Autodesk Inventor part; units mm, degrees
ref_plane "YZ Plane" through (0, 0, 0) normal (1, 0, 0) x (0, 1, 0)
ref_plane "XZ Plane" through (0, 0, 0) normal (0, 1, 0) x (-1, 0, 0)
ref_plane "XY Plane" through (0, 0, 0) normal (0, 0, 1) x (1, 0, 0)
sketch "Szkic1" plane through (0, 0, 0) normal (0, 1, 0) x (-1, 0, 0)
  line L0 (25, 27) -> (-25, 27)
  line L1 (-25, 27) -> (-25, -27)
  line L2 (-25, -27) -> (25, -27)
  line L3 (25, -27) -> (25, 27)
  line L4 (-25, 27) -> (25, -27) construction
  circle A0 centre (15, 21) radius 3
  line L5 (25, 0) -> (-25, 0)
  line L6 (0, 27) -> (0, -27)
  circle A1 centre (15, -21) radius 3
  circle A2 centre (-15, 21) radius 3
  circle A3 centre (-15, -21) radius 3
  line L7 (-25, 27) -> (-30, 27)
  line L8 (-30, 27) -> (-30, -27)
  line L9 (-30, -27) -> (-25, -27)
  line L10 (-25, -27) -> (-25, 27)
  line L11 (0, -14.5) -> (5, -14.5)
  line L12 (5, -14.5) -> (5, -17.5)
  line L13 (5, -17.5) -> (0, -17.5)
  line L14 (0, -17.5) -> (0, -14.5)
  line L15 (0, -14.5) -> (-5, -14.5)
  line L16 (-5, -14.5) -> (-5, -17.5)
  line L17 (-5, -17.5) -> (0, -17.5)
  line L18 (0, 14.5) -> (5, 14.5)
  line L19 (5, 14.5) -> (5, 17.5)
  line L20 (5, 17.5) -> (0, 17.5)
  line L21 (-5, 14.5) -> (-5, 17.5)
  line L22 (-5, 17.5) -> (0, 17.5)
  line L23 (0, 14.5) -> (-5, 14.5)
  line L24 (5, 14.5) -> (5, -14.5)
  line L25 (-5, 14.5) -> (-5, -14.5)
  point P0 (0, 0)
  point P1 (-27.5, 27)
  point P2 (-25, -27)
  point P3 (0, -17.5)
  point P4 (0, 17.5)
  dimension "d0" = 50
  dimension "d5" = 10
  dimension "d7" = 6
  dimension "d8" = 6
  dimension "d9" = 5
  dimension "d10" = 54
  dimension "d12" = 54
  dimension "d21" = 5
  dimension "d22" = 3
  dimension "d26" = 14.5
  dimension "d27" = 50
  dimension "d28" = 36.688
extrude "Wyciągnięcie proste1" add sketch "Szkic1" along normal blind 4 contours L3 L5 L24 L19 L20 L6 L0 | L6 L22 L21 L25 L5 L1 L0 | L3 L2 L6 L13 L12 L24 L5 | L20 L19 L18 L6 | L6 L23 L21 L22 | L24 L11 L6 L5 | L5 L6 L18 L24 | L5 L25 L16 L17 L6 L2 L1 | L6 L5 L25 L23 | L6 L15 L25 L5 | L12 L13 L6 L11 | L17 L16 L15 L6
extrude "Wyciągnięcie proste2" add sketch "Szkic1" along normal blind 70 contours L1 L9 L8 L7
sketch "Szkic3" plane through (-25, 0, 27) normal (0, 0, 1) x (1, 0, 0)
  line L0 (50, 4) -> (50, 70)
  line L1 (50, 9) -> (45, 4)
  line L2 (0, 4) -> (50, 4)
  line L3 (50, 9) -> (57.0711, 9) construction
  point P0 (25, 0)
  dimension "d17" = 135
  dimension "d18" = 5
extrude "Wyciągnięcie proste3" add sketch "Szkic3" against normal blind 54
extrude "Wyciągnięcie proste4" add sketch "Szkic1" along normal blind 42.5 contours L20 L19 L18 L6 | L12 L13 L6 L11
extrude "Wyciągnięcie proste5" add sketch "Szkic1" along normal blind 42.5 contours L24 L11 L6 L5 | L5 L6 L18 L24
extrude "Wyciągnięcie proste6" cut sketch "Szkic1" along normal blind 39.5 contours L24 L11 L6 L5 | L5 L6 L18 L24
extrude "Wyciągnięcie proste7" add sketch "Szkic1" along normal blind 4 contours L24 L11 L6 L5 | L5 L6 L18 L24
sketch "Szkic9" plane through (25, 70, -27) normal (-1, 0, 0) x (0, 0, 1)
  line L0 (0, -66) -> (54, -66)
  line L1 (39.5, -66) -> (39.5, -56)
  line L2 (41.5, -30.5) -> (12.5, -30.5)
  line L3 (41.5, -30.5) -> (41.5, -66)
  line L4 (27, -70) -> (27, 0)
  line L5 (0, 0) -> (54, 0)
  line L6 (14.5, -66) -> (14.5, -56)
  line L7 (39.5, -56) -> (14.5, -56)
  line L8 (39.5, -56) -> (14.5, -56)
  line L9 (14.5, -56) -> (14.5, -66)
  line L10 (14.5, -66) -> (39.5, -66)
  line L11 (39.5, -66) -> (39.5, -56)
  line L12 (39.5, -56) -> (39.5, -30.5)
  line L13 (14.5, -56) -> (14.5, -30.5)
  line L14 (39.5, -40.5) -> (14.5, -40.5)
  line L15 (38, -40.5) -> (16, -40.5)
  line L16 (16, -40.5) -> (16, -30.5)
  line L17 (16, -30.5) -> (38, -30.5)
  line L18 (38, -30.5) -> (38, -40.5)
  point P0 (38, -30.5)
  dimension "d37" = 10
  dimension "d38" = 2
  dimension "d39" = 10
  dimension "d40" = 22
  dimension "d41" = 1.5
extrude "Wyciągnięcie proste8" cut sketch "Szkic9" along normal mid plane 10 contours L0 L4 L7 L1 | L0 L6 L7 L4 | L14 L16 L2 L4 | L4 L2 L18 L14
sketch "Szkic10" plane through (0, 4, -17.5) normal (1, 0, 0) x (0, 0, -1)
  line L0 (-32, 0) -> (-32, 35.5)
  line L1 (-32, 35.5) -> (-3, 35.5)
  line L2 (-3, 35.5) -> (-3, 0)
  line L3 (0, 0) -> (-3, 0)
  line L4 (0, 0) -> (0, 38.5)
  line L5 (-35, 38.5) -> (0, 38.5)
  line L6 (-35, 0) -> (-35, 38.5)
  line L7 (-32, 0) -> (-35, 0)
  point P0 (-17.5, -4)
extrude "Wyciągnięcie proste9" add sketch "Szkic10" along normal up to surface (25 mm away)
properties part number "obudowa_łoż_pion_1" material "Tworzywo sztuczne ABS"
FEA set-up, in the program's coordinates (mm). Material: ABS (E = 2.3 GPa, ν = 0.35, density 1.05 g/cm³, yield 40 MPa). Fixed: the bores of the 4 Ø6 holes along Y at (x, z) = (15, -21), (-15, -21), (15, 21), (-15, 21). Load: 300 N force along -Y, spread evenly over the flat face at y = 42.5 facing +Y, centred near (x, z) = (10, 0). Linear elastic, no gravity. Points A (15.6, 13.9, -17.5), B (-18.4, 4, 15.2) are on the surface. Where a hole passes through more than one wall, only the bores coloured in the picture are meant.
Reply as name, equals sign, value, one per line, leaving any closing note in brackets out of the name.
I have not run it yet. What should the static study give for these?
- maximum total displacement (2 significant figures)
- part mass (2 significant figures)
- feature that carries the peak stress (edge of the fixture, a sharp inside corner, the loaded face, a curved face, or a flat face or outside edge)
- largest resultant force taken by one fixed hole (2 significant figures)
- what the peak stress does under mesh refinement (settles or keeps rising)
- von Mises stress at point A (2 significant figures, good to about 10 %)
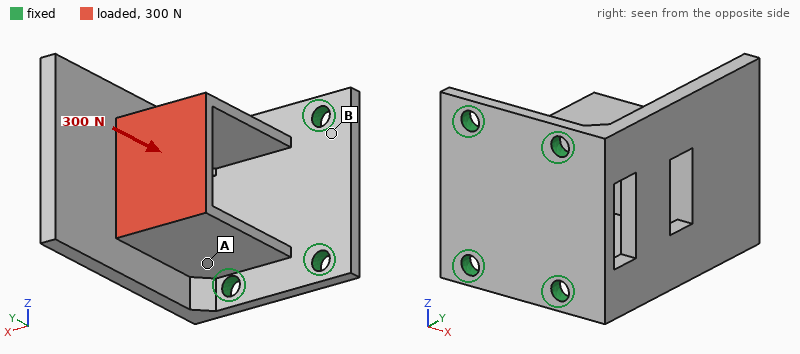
maximum total displacement = 0.38 mm
part mass = 39 g
feature that carries the peak stress = edge of the fixture
largest resultant force taken by one fixed hole = 120 N
what the peak stress does under mesh refinement = keeps rising
von Mises stress at point A = 2.3 MPa
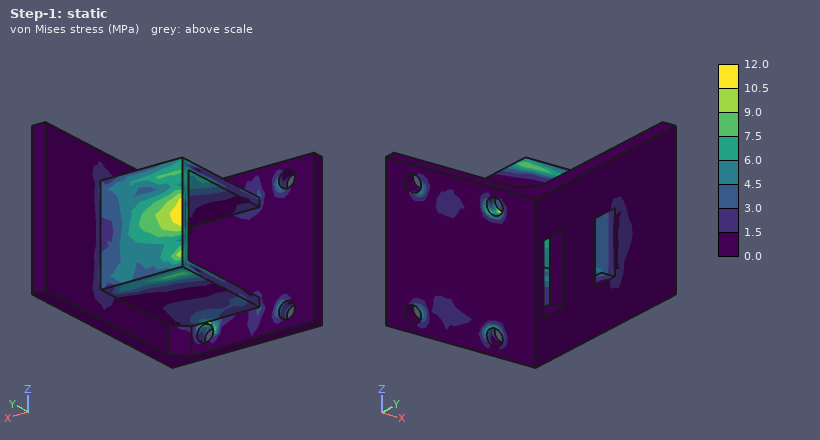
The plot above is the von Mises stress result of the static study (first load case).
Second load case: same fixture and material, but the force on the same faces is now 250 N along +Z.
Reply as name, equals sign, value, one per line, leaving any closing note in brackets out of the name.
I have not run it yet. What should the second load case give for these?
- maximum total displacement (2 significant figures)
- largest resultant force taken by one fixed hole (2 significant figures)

maximum total displacement = 1.2 mm
largest resultant force taken by one fixed hole = 330 N
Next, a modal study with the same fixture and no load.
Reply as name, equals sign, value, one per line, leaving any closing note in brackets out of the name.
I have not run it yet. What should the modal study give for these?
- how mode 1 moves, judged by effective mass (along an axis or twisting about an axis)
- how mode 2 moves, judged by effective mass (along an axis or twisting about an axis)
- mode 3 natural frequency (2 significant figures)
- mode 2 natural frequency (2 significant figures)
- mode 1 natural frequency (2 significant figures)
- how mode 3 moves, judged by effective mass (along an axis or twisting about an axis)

how mode 1 moves, judged by effective mass = along X
how mode 2 moves, judged by effective mass = along Z
mode 3 natural frequency = 1400 Hz
mode 2 natural frequency = 740 Hz
mode 1 natural frequency = 650 Hz
how mode 3 moves, judged by effective mass = along Z
